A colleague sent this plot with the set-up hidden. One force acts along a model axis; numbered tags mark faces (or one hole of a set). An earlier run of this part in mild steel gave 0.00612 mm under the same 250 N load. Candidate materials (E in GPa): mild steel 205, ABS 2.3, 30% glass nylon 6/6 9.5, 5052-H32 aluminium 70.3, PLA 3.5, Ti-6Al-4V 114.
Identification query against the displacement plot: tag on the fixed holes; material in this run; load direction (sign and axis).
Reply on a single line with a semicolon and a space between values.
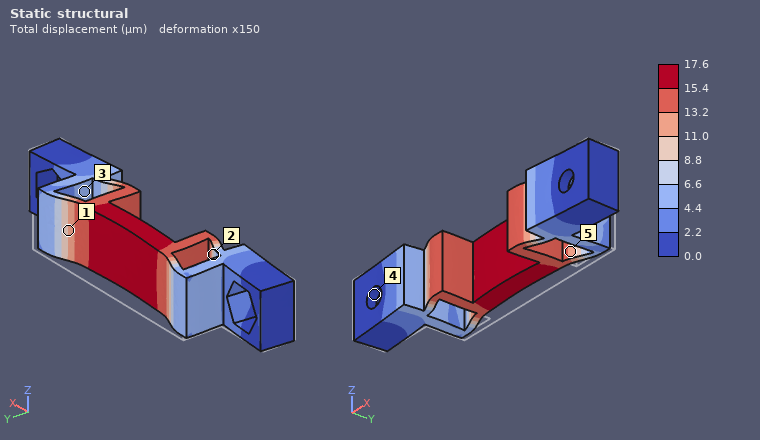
4; 5052-H32 aluminium; -Y
